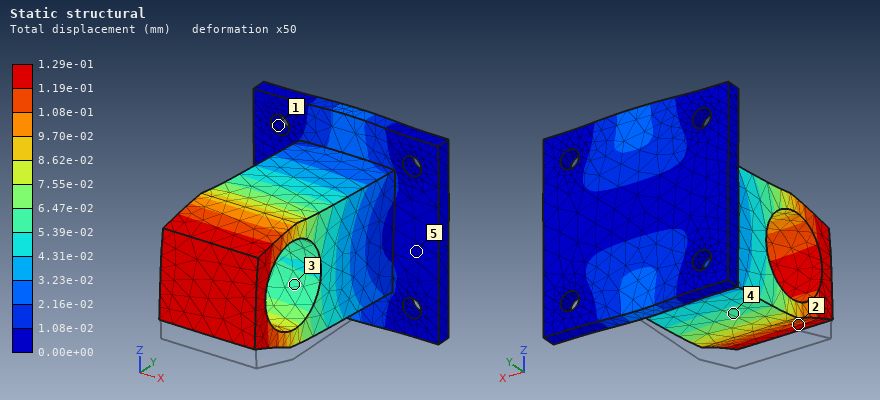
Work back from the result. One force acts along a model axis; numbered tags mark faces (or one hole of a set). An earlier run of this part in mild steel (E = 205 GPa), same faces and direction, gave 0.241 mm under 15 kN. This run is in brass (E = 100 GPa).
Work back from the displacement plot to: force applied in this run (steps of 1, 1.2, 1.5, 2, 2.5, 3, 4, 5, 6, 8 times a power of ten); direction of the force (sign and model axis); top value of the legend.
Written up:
4 kN
+Z
1.29e-01 mm
